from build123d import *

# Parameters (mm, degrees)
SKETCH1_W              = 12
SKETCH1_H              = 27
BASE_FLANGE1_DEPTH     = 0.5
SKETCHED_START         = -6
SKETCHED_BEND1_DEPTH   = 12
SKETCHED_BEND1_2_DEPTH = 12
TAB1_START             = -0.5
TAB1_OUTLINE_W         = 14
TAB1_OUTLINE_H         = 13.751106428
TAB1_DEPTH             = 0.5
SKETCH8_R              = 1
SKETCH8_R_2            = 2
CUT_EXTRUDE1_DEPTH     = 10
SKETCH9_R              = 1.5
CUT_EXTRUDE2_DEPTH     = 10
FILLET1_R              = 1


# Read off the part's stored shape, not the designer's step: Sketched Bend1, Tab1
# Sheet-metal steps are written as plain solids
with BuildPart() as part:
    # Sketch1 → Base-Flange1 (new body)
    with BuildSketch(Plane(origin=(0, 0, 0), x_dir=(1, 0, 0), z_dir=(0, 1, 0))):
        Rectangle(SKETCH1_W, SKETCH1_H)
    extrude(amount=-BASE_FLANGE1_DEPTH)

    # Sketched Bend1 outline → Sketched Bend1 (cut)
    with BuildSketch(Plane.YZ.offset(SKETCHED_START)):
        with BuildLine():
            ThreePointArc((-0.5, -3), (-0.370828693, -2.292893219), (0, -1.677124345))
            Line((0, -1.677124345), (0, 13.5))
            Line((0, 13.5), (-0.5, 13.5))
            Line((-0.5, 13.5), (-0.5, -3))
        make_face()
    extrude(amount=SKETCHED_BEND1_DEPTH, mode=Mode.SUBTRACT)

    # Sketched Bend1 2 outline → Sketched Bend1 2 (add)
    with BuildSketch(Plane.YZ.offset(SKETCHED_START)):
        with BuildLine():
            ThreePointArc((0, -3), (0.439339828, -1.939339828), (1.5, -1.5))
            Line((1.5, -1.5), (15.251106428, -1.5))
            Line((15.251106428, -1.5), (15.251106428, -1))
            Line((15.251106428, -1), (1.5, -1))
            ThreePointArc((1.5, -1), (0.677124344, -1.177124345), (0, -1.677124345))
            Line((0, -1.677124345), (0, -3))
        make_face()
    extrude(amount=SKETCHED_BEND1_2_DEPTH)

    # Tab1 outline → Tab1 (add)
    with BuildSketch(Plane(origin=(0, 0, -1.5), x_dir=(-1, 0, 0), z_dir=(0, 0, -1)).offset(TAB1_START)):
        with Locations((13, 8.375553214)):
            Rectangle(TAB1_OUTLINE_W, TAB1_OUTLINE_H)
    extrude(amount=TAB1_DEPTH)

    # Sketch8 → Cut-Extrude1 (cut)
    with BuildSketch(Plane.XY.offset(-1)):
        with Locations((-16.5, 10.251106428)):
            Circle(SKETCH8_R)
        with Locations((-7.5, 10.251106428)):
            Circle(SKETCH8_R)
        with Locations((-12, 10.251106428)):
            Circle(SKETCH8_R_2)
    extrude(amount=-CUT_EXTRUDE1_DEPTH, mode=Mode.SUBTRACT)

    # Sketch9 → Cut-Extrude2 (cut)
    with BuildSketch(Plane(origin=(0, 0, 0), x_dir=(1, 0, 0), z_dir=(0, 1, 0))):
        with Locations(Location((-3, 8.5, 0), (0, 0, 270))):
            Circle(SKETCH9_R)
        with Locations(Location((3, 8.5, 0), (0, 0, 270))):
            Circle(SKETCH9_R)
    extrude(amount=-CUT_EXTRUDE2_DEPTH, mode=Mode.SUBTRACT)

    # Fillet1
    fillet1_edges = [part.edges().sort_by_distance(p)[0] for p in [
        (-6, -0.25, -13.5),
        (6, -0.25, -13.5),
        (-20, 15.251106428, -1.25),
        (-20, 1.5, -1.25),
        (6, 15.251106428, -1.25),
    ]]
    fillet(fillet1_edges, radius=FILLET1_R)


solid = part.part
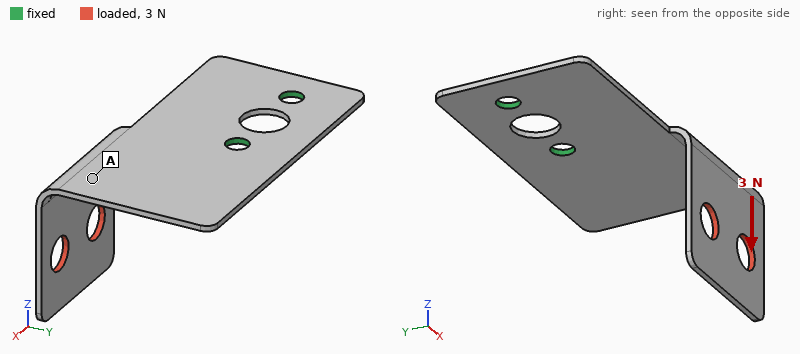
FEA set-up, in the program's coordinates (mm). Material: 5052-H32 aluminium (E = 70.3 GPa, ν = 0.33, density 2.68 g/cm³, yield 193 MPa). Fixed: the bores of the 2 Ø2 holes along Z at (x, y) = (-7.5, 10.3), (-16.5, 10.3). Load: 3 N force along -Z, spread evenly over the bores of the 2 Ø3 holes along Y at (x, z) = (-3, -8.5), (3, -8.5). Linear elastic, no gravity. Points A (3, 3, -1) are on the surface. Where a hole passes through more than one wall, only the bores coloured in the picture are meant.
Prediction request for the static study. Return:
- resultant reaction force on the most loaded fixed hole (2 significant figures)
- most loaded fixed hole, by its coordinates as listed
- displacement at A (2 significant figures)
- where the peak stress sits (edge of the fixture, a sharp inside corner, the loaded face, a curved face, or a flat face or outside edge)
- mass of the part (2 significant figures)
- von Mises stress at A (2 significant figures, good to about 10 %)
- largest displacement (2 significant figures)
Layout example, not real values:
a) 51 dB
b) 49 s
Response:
a) 3.7 N
b) (-7.5, 10.3)
c) 0.17 mm
d) a flat face or outside edge
e) 0.65 g
f) 13 MPa
g) 0.37 mm
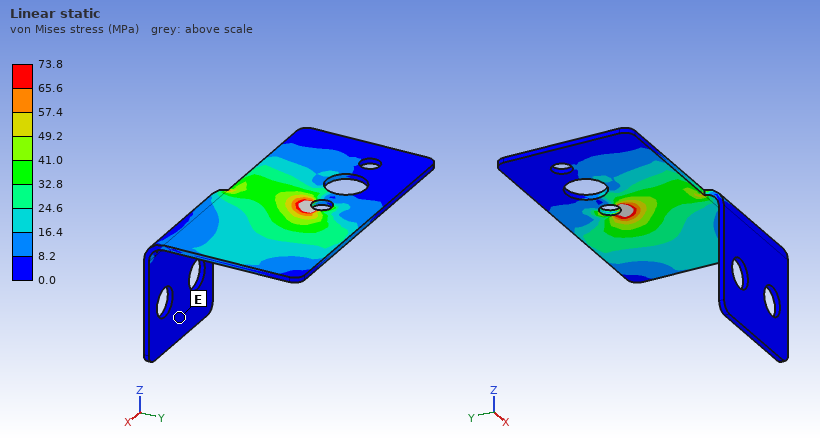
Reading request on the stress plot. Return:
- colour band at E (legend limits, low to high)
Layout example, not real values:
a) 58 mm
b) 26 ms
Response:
a) 0.0 to 8.2 MPa
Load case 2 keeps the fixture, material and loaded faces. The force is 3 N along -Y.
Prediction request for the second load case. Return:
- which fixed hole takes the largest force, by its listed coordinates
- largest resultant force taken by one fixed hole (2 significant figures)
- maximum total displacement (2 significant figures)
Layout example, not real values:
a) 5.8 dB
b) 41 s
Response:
a) (-7.5, 10.3)
b) 4.8 N
c) 0.38 mm
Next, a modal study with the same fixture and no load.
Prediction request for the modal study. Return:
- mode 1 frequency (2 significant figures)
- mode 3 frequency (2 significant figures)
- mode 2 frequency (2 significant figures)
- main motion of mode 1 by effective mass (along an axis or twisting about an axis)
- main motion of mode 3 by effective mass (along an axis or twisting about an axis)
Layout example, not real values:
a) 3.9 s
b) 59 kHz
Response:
a) 1000 Hz
b) 3200 Hz
c) 1600 Hz
d) along Z
e) along Z
